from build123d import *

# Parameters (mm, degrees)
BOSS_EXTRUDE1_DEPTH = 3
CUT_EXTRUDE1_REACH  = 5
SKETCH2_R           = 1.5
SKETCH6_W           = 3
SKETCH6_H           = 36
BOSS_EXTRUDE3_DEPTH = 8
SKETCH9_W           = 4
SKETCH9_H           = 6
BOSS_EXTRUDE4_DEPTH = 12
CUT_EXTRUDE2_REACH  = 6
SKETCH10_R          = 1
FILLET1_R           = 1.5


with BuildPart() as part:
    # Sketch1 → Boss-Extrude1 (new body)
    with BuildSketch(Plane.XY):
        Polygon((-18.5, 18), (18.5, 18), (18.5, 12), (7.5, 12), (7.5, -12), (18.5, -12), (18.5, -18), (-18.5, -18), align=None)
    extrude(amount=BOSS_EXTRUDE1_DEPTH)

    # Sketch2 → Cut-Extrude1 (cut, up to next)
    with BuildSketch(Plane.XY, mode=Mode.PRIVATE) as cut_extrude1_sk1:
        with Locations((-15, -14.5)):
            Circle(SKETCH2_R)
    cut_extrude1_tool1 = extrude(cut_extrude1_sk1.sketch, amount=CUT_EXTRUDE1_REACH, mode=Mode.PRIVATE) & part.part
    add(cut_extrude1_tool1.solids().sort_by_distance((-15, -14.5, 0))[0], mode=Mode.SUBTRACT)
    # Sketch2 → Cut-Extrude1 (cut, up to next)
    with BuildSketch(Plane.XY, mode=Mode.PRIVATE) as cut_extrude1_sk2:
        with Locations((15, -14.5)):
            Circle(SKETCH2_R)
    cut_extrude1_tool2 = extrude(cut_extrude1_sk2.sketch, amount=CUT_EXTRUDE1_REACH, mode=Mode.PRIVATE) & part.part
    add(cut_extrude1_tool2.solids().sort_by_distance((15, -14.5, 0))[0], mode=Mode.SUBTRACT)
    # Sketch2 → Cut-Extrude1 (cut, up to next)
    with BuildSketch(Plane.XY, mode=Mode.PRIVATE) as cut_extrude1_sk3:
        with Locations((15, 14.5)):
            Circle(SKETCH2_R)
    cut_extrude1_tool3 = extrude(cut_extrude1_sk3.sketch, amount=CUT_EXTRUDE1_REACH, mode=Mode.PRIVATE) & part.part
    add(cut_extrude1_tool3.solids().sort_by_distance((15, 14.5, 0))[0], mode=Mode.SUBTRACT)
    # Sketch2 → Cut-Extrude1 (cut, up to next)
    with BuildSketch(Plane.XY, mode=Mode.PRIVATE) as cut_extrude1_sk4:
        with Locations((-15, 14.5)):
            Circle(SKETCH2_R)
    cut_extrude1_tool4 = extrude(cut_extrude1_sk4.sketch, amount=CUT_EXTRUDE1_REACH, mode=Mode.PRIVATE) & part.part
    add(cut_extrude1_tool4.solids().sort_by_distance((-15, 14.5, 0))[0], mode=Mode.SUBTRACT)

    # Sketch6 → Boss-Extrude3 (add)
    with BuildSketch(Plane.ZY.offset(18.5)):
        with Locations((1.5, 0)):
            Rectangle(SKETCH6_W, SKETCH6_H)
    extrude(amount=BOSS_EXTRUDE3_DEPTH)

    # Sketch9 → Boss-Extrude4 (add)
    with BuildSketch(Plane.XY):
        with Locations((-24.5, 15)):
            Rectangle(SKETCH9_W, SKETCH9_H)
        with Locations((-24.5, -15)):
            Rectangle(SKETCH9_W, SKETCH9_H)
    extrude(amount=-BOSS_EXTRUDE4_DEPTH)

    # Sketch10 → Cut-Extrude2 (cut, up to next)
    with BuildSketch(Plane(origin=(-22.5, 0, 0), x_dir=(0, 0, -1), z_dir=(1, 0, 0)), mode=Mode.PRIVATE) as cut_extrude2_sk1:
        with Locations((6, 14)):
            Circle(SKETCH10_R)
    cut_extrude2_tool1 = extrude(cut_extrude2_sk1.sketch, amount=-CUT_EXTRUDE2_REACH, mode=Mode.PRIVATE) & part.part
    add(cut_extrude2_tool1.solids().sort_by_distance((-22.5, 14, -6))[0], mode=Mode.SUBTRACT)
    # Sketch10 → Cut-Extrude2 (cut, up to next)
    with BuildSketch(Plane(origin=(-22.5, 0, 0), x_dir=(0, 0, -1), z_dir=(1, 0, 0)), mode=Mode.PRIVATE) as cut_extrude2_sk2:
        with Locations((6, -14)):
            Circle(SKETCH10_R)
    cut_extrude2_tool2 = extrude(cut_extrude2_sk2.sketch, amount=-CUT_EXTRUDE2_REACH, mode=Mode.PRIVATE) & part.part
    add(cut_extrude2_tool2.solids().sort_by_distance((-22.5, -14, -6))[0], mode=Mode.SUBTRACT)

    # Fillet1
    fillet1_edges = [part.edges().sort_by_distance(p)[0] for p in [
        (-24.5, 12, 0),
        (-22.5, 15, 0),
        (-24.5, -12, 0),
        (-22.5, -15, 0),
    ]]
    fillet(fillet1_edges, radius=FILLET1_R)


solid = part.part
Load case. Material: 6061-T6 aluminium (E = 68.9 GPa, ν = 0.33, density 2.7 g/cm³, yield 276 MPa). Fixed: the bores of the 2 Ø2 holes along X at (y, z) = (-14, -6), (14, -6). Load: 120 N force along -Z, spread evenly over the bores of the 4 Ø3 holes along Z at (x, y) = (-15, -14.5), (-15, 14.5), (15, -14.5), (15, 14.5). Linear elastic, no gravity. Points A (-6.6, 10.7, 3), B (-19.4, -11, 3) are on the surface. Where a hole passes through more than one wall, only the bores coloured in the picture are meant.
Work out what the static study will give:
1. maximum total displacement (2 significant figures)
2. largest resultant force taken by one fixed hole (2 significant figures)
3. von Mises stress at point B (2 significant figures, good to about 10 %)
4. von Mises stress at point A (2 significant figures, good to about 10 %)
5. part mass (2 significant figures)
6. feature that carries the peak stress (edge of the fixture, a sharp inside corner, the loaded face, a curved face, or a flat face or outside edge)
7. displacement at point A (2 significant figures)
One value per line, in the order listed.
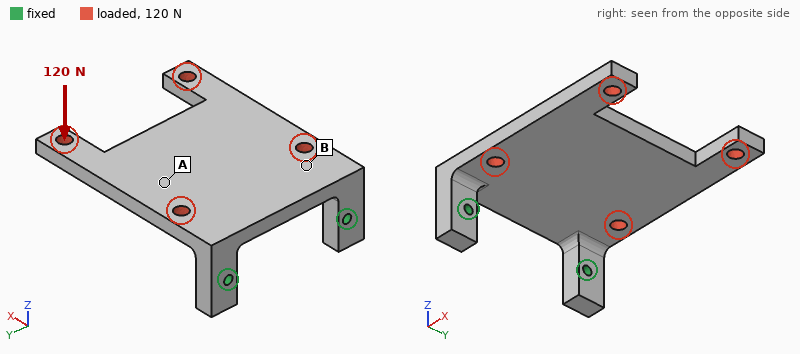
0.51 mm
62 N
48 MPa
24 MPa
12 g
a curved face
0.16 mm
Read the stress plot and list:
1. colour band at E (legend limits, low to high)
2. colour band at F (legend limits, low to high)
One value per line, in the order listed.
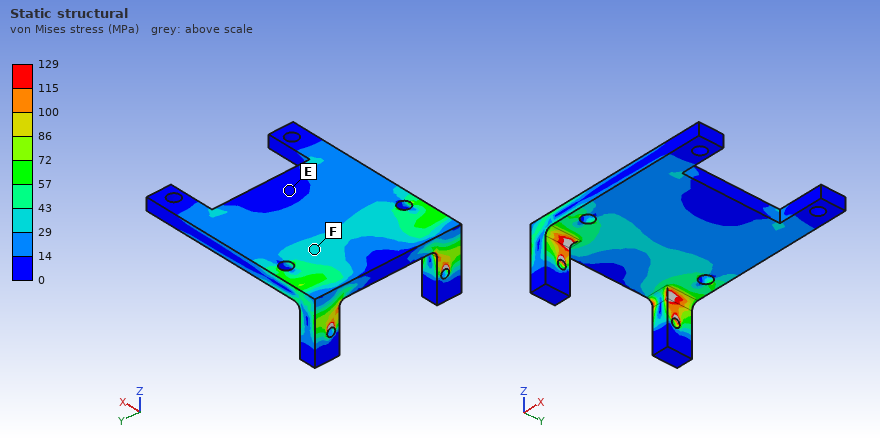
0 to 14 MPa
29 to 43 MPa
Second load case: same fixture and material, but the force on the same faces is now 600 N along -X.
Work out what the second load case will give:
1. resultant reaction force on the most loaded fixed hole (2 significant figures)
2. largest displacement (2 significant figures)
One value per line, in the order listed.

300 N
0.17 mm
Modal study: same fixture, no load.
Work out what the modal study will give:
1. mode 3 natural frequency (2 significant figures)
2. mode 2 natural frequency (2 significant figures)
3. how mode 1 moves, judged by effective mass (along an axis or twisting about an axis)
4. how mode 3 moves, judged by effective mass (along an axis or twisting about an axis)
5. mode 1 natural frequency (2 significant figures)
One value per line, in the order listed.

5500 Hz
3400 Hz
along Z
along Y
1300 Hz
